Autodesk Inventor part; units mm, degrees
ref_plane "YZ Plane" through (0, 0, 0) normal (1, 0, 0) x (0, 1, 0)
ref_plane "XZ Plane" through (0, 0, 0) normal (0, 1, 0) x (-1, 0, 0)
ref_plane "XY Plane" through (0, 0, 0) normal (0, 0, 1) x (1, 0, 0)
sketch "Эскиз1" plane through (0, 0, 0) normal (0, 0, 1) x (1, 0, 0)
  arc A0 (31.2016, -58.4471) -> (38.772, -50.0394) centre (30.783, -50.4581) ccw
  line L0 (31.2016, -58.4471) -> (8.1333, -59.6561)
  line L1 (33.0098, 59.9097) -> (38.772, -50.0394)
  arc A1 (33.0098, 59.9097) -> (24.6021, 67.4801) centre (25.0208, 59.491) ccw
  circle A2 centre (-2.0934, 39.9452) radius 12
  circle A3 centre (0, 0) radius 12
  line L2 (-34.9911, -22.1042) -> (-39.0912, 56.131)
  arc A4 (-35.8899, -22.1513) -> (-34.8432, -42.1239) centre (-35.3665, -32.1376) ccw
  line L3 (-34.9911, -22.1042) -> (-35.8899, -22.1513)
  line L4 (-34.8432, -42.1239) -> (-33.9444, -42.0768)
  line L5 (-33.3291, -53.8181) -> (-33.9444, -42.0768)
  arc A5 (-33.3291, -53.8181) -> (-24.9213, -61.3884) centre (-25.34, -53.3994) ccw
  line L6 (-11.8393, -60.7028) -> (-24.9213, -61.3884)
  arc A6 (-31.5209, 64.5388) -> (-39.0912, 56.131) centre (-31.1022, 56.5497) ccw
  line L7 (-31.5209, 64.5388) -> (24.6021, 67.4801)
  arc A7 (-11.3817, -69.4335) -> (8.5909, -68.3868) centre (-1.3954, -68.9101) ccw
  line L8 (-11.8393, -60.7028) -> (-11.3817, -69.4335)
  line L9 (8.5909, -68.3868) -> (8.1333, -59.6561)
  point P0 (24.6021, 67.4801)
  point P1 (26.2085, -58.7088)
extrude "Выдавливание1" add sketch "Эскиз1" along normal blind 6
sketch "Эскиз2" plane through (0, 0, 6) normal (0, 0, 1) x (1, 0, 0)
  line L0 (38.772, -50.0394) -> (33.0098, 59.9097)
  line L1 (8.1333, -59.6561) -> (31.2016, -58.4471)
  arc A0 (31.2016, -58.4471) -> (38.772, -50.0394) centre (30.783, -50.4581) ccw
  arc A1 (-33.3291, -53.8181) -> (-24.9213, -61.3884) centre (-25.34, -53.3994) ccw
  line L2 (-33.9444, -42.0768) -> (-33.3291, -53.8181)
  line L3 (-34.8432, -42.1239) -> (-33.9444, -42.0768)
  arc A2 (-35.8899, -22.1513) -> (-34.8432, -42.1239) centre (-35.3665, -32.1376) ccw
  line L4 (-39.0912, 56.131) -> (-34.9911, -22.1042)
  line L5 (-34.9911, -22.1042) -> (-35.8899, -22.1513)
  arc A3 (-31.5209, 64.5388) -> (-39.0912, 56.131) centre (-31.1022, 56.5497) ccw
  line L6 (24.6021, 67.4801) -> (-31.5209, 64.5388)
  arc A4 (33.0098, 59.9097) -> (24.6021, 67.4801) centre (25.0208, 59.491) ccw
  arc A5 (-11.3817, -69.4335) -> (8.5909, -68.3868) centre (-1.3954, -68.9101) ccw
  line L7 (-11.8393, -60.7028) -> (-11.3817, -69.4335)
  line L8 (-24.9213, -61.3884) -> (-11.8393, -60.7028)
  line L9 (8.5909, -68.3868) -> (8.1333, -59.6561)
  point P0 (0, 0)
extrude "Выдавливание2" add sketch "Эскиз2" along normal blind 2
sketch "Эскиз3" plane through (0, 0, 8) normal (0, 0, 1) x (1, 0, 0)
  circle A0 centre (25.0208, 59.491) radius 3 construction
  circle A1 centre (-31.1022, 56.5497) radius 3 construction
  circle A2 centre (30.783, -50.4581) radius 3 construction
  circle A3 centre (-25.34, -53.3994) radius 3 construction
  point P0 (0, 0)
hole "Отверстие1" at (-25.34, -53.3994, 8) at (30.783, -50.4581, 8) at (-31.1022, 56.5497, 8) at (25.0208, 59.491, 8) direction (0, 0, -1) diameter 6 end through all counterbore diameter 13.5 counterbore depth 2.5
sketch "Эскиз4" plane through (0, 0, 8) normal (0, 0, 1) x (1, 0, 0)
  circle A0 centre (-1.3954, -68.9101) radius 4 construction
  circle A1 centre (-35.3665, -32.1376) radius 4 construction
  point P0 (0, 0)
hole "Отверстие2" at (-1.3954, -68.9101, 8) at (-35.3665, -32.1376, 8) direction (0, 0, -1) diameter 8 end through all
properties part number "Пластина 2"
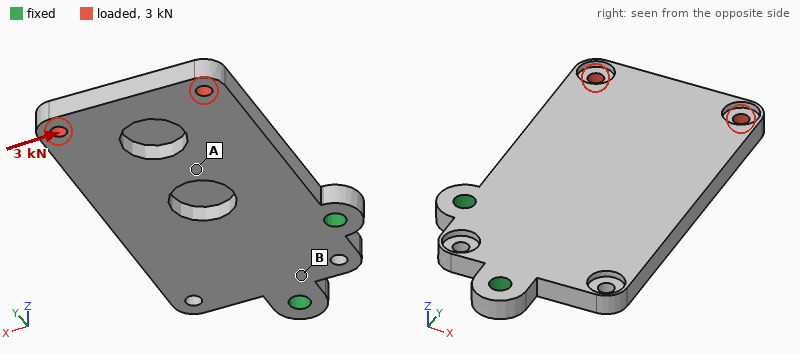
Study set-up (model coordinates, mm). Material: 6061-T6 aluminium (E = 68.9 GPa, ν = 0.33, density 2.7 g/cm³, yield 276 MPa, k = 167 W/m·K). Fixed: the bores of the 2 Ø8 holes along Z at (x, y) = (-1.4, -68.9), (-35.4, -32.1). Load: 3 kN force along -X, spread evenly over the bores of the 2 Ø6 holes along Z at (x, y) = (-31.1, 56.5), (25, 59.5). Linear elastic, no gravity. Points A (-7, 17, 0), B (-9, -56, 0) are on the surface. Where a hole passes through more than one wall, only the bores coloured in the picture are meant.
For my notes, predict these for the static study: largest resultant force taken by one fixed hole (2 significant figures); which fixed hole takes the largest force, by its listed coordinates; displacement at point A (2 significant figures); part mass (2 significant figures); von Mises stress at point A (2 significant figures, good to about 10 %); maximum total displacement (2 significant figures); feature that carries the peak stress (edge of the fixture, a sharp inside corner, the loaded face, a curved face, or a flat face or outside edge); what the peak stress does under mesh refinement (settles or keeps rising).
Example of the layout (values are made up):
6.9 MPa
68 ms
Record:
7.5 kN
(-35.4, -32.1)
0.080 mm
180 g
28 MPa
0.21 mm
a sharp inside corner
keeps rising
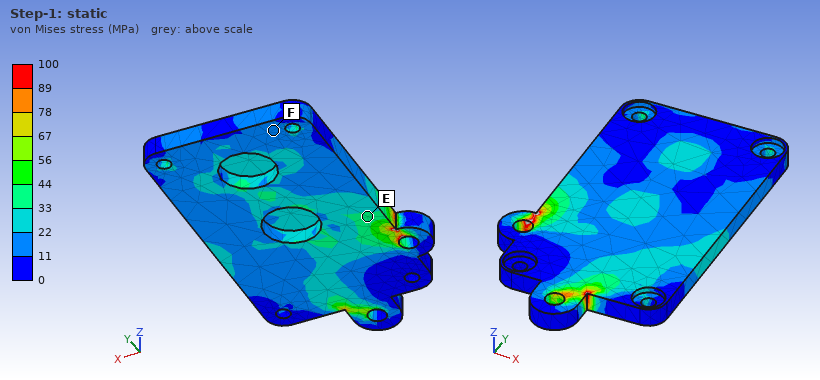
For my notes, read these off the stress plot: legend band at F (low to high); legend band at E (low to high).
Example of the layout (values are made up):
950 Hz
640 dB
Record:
11 to 22 MPa
33 to 44 MPa
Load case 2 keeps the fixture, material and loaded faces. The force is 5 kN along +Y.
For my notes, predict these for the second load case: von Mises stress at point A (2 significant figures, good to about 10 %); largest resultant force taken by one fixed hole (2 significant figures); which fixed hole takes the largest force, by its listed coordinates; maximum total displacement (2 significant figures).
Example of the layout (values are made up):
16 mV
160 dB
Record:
8.5 MPa
3.6 kN
(-1.4, -68.9)
0.25 mm
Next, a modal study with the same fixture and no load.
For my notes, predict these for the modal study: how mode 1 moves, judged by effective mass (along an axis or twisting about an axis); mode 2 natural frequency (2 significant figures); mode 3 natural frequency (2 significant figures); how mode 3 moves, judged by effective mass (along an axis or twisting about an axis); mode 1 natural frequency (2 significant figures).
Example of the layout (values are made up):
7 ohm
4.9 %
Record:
along Z
1400 Hz
2700 Hz
along Z
520 Hz
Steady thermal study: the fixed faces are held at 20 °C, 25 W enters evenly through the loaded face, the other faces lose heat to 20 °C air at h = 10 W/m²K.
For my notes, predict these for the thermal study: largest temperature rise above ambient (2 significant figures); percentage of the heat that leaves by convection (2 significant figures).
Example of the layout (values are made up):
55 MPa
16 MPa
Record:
35 K
14 %
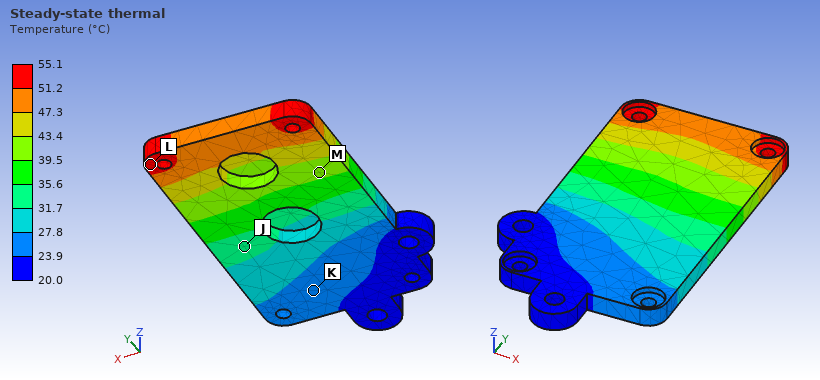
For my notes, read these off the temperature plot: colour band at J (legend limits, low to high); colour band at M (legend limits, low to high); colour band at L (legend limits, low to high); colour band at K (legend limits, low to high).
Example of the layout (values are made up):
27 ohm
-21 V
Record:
31.7 to 35.6 °C
39.5 to 43.4 °C
51.2 to 55.1 °C
23.9 to 27.8 °C
